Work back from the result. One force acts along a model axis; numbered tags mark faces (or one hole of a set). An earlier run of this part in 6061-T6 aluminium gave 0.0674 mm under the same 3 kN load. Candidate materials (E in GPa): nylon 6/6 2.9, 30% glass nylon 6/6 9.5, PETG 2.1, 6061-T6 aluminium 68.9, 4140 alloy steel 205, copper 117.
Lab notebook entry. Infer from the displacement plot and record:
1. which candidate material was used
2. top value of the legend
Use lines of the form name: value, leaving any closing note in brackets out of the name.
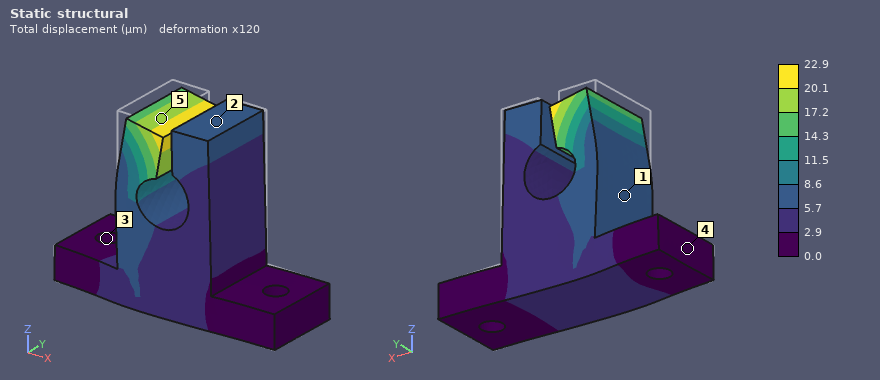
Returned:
which candidate material was used: 4140 alloy steel
top value of the legend: 22.9 µm
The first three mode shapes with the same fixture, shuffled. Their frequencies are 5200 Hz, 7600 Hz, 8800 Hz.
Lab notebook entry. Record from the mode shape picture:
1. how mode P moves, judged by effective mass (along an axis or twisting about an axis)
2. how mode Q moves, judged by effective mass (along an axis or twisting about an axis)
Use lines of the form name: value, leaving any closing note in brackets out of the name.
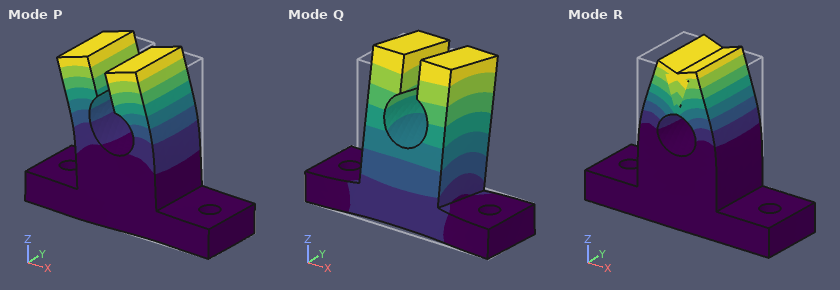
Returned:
how mode P moves, judged by effective mass: along X
how mode Q moves, judged by effective mass: along Y
